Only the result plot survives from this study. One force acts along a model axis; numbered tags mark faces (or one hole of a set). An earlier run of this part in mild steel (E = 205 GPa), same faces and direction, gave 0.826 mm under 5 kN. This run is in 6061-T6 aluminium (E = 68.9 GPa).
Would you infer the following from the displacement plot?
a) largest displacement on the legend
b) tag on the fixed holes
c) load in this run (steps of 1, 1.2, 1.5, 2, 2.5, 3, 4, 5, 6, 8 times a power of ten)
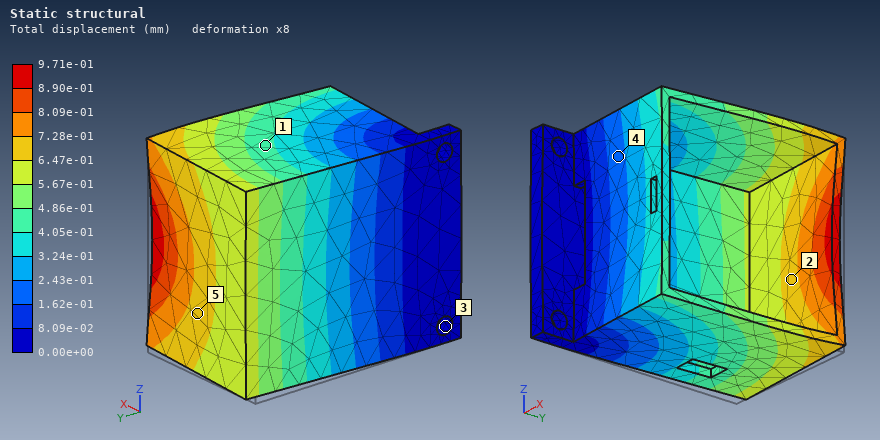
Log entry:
9.71e-01 mm
3
2 kN
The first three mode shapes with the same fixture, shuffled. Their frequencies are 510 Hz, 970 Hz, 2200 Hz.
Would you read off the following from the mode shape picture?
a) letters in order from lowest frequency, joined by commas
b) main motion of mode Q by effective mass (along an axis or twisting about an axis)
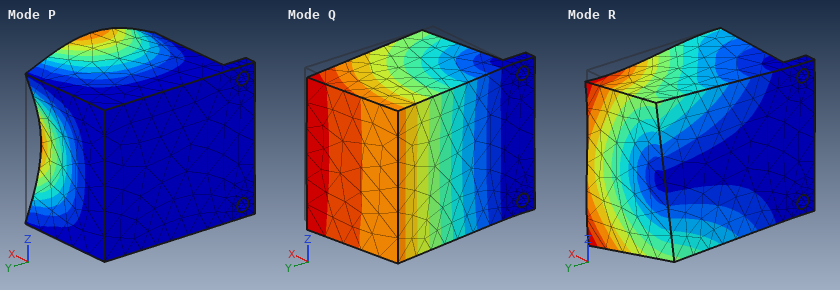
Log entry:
Q, R, P
along X
